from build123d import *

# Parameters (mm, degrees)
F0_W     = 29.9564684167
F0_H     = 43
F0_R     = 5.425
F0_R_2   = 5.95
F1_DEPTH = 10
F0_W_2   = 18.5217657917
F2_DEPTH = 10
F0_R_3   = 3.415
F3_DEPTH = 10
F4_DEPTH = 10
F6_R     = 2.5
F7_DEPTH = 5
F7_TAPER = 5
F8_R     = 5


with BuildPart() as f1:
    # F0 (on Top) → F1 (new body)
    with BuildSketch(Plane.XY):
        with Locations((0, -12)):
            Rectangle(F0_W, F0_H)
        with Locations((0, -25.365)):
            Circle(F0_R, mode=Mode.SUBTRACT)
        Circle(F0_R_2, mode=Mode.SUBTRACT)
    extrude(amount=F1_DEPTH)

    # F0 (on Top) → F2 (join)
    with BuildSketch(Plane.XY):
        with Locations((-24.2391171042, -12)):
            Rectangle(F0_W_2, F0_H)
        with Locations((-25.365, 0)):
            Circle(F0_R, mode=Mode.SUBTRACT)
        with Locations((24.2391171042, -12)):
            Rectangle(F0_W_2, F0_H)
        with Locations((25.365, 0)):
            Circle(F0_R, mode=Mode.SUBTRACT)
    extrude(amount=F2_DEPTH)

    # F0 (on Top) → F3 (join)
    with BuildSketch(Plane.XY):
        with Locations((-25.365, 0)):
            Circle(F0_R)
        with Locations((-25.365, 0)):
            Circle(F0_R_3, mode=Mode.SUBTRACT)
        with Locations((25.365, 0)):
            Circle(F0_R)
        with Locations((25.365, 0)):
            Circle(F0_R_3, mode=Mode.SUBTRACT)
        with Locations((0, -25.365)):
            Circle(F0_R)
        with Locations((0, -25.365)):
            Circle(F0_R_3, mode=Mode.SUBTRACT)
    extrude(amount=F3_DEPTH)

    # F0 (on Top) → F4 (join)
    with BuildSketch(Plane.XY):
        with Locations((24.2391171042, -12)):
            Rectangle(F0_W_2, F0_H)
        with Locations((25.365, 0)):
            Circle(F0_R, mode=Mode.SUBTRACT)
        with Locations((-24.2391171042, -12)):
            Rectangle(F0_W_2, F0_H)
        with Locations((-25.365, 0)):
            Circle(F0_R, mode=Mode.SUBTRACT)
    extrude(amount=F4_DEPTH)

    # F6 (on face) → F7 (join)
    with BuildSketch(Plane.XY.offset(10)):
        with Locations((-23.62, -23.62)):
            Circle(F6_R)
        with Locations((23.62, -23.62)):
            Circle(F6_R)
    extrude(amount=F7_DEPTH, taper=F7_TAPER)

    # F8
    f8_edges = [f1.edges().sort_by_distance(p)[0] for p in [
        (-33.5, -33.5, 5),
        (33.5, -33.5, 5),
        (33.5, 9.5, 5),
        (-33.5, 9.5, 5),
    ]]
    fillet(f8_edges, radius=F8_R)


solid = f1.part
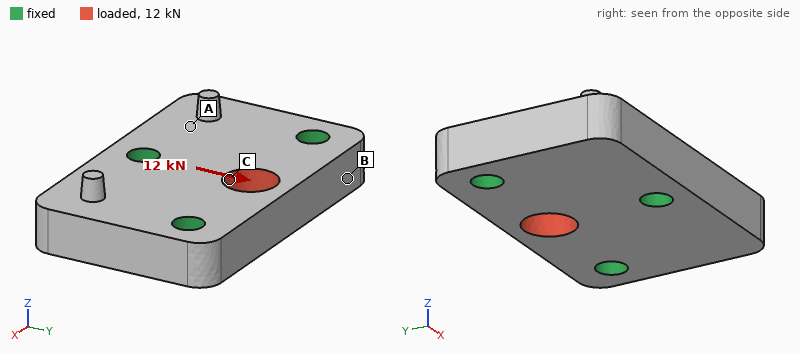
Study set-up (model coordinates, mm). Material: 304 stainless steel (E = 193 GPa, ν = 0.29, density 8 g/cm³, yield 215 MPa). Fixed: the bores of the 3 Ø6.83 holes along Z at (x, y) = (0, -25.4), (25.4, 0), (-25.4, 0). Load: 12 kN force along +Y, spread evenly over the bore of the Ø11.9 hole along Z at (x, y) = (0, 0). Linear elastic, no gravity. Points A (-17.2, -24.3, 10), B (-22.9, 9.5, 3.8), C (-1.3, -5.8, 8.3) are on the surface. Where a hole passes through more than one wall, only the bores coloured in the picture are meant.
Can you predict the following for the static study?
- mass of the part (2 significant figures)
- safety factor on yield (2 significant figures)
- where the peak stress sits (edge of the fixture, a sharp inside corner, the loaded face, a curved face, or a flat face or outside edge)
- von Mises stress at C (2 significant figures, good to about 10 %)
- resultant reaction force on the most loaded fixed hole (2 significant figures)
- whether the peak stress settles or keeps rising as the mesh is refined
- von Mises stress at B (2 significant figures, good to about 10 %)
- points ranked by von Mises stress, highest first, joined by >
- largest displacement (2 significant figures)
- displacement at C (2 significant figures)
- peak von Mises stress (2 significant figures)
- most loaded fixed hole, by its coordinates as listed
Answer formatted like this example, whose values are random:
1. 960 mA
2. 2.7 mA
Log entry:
1. 210 g
2. 1.8
3. a flat face or outside edge
4. 41 MPa
5. 6.4 kN
6. settles
7. 19 MPa
8. C > B > A
9. 11 µm
10. 3.6 µm
11. 120 MPa
12. (0, -25.4)
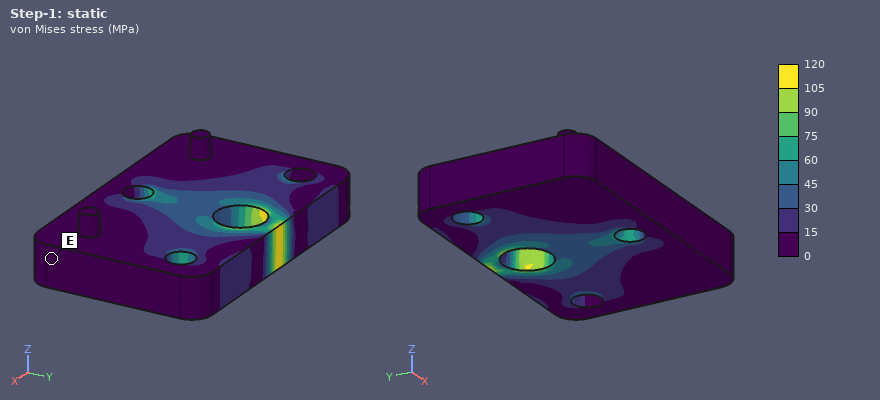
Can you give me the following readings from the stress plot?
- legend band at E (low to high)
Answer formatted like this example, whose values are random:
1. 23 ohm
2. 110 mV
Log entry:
1. 0 to 15 MPa
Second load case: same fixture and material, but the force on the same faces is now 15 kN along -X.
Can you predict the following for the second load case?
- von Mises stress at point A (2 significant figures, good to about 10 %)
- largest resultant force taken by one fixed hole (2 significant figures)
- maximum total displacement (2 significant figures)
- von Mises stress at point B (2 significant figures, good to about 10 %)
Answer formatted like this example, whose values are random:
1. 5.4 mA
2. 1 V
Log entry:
1. 6.1 MPa
2. 6.3 kN
3. 5.3 µm
4. 16 MPa
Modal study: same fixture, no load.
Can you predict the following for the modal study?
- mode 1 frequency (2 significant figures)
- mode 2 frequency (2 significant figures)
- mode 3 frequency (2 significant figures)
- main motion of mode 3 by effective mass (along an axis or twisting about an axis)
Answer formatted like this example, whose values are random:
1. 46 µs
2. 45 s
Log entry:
1. 13 kHz
2. 13 kHz
3. 21 kHz
4. along Z
